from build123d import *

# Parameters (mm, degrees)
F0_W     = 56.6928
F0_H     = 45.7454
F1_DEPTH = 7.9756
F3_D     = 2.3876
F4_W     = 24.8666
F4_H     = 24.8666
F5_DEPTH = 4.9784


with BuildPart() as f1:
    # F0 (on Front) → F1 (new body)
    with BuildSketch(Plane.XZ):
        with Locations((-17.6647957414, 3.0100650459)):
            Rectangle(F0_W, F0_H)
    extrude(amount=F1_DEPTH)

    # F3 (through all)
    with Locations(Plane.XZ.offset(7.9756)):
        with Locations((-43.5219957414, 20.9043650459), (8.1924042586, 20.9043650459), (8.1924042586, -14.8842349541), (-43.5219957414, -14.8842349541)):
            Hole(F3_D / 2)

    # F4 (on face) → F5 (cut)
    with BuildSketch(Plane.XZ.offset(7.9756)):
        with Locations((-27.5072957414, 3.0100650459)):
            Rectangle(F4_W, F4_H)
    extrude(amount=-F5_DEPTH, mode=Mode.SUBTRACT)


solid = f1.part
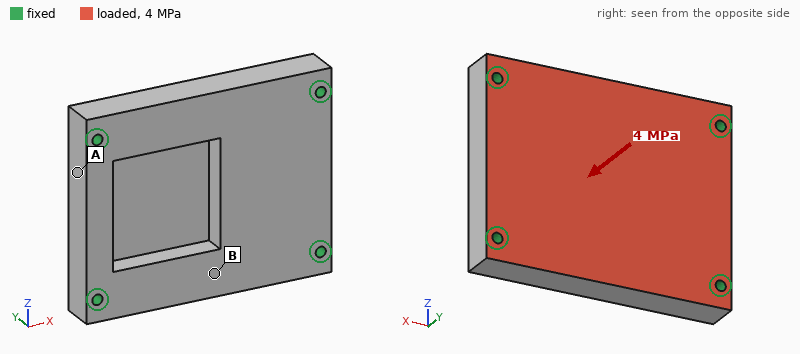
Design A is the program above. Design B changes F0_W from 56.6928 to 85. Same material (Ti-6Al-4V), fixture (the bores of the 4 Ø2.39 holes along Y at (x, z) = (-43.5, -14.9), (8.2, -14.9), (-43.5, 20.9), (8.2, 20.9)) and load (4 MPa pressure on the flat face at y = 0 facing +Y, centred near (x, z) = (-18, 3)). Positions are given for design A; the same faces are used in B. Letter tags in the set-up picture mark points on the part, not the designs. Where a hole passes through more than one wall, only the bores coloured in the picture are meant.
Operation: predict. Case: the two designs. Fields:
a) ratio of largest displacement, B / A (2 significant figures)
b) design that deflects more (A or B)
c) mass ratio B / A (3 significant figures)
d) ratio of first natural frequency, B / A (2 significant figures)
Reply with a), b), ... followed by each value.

a) 0.85
b) A
c) 1.59
d) 1.0
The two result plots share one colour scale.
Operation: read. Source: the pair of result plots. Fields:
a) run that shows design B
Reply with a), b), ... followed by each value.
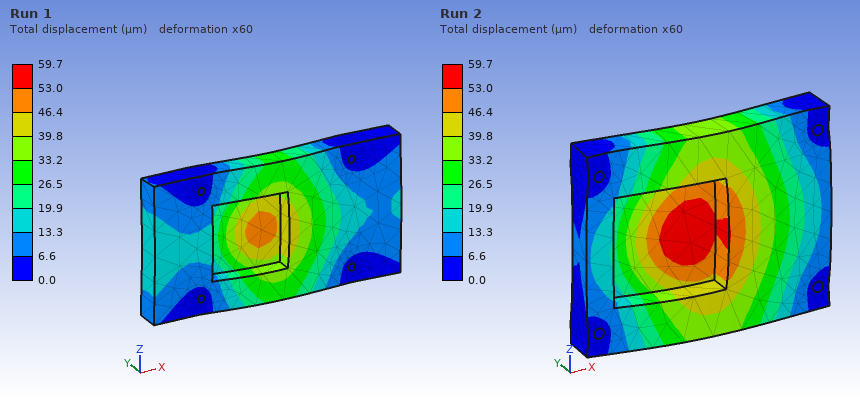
a) Run 1
